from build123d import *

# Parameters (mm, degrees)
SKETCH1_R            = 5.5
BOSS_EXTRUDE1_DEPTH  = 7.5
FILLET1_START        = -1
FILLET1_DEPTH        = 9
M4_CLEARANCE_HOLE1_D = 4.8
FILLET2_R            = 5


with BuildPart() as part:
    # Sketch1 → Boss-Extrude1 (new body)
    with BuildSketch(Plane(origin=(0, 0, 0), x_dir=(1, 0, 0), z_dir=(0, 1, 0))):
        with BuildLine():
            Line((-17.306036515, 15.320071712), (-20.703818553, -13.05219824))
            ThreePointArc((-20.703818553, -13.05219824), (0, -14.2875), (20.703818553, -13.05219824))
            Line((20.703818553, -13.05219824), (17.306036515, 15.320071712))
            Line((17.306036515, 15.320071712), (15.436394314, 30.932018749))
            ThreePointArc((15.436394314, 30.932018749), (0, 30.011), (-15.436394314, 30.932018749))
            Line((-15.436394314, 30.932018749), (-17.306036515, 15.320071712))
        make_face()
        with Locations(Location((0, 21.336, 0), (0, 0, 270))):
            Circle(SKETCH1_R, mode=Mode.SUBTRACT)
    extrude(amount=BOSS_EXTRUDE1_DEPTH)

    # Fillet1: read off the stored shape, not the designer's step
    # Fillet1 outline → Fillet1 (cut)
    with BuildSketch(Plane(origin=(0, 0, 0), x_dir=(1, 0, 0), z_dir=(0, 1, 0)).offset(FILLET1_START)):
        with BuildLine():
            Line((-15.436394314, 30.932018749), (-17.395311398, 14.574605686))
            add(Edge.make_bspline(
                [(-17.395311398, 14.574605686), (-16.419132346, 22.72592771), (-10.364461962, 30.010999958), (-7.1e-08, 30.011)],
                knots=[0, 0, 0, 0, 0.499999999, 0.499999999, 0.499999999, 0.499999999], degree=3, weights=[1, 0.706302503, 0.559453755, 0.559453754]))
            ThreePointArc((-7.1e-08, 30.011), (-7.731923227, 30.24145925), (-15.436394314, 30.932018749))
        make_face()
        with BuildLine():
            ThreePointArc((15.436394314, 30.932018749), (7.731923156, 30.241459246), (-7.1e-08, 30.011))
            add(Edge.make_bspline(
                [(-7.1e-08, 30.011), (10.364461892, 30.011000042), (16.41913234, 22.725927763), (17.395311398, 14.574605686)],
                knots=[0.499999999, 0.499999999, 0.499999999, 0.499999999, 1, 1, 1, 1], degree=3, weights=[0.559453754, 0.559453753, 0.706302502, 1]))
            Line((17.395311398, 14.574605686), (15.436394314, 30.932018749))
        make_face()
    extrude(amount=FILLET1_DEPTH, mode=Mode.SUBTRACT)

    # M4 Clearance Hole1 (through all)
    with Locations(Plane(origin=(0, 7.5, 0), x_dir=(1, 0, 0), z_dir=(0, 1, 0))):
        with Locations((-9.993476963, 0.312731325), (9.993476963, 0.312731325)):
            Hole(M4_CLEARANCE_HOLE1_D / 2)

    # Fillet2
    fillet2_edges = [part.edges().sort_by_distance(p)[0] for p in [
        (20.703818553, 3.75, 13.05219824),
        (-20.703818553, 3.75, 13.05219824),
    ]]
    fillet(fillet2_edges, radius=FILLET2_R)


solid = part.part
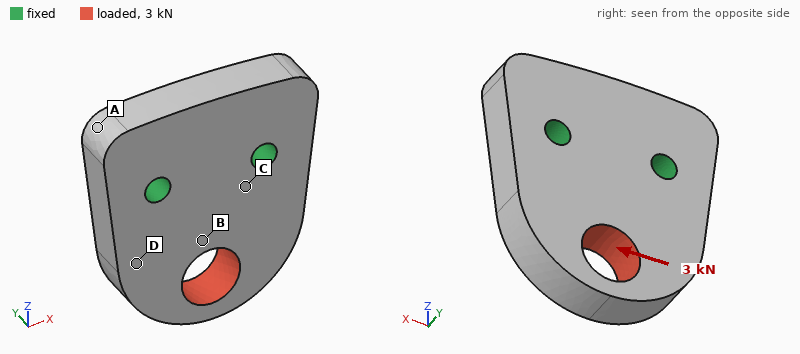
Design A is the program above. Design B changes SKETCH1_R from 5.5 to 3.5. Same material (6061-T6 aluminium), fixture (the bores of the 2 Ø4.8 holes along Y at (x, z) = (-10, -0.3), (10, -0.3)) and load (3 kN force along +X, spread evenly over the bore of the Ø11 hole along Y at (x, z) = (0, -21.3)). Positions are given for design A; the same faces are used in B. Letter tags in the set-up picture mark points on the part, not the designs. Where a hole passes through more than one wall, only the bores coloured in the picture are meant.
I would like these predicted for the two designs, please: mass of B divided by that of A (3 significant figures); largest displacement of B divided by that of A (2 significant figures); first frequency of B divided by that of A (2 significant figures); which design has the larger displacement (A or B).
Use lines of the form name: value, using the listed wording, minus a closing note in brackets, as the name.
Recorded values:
mass of B divided by that of A: 1.04
largest displacement of B divided by that of A: 0.76
first frequency of B divided by that of A: 0.94
which design has the larger displacement: A
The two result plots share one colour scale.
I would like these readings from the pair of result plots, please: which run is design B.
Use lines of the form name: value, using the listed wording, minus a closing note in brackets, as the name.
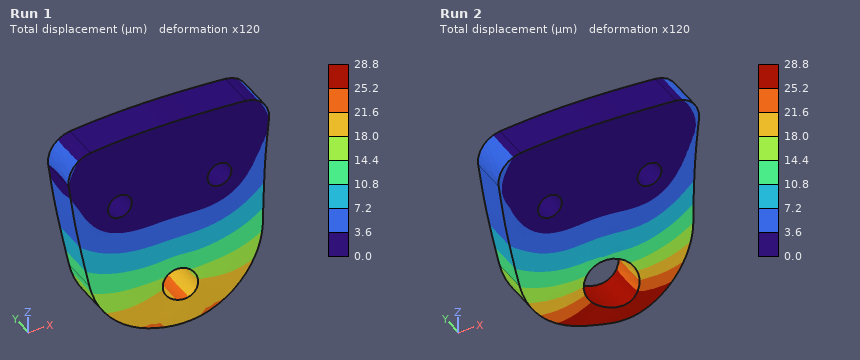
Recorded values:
which run is design B: Run 1
